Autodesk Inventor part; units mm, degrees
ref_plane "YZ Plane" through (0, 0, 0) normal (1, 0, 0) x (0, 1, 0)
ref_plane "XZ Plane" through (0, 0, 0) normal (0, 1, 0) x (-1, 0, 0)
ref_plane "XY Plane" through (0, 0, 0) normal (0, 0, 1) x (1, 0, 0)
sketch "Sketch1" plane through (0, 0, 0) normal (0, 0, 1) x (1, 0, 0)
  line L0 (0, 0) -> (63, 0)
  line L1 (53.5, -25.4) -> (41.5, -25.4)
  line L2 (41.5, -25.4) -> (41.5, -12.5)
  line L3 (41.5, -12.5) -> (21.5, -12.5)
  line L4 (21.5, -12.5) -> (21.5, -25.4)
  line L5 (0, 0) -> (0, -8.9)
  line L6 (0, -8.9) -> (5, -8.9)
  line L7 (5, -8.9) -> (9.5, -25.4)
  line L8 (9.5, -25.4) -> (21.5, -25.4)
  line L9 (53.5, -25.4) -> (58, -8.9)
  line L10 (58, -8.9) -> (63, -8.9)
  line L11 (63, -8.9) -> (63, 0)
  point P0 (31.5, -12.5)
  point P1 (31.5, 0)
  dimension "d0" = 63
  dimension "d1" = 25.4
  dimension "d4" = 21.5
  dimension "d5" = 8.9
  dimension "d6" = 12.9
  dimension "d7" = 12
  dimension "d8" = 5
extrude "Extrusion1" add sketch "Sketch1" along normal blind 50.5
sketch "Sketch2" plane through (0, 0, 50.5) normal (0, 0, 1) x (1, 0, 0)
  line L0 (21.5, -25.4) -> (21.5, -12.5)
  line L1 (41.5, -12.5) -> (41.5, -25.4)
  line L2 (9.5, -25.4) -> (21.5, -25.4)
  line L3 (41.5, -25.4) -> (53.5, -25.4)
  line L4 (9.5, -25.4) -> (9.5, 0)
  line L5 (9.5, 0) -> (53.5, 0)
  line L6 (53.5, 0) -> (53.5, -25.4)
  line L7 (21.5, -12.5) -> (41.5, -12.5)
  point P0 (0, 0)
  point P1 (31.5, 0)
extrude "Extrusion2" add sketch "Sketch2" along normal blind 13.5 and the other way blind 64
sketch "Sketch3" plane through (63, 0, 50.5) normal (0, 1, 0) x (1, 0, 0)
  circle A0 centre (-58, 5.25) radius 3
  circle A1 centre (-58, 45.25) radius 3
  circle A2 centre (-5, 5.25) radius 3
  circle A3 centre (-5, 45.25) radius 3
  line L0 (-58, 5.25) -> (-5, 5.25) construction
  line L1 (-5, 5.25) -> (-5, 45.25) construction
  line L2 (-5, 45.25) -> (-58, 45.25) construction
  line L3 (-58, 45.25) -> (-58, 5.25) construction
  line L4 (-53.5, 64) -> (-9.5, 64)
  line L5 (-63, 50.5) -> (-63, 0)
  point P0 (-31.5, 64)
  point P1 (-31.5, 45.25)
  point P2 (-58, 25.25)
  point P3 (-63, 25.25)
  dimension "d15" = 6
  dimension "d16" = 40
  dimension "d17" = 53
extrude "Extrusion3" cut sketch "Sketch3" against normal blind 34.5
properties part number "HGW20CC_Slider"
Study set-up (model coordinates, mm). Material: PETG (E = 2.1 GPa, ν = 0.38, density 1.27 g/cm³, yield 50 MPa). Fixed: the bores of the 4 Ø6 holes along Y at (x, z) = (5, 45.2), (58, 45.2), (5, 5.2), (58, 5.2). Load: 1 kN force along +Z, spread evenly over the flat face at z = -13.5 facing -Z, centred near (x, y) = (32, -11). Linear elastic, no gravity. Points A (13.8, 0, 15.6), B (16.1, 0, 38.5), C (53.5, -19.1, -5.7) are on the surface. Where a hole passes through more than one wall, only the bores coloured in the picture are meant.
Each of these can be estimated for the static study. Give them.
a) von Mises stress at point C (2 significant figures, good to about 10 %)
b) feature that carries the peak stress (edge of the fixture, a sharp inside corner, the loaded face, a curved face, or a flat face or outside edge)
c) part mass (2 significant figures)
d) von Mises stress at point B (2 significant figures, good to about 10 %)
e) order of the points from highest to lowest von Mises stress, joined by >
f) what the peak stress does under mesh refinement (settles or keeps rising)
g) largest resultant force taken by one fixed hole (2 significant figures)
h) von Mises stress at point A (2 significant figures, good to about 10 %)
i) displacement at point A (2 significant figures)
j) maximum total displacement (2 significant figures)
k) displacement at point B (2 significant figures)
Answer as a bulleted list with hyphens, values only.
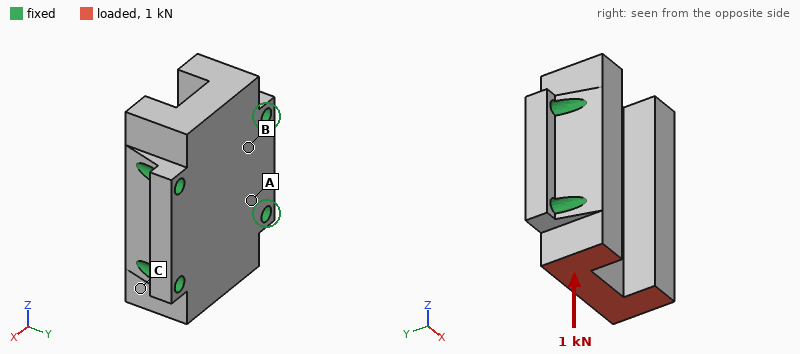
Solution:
- 1.4 MPa
- edge of the fixture
- 99 g
- 0.47 MPa
- C > A > B
- keeps rising
- 330 N
- 0.81 MPa
- 7.5 µm
- 28 µm
- 4.6 µm
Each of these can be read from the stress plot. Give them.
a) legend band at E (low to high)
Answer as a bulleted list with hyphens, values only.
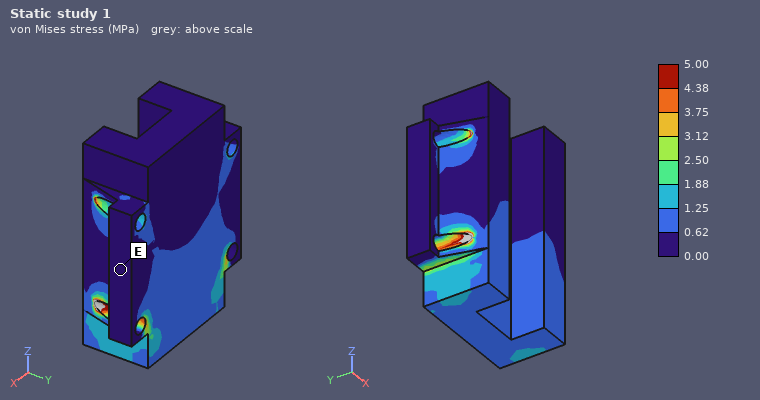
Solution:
- 0.00 to 0.62 MPa
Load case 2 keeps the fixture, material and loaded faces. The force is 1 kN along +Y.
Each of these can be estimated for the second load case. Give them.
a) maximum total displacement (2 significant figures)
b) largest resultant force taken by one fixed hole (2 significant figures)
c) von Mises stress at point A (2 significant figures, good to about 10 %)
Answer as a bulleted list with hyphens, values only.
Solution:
- 0.19 mm
- 620 N
- 2.7 MPa
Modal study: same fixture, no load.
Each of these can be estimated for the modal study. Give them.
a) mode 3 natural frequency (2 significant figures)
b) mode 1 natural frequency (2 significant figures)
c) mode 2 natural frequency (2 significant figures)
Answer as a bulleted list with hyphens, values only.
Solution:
- 5200 Hz
- 3600 Hz
- 3800 Hz
